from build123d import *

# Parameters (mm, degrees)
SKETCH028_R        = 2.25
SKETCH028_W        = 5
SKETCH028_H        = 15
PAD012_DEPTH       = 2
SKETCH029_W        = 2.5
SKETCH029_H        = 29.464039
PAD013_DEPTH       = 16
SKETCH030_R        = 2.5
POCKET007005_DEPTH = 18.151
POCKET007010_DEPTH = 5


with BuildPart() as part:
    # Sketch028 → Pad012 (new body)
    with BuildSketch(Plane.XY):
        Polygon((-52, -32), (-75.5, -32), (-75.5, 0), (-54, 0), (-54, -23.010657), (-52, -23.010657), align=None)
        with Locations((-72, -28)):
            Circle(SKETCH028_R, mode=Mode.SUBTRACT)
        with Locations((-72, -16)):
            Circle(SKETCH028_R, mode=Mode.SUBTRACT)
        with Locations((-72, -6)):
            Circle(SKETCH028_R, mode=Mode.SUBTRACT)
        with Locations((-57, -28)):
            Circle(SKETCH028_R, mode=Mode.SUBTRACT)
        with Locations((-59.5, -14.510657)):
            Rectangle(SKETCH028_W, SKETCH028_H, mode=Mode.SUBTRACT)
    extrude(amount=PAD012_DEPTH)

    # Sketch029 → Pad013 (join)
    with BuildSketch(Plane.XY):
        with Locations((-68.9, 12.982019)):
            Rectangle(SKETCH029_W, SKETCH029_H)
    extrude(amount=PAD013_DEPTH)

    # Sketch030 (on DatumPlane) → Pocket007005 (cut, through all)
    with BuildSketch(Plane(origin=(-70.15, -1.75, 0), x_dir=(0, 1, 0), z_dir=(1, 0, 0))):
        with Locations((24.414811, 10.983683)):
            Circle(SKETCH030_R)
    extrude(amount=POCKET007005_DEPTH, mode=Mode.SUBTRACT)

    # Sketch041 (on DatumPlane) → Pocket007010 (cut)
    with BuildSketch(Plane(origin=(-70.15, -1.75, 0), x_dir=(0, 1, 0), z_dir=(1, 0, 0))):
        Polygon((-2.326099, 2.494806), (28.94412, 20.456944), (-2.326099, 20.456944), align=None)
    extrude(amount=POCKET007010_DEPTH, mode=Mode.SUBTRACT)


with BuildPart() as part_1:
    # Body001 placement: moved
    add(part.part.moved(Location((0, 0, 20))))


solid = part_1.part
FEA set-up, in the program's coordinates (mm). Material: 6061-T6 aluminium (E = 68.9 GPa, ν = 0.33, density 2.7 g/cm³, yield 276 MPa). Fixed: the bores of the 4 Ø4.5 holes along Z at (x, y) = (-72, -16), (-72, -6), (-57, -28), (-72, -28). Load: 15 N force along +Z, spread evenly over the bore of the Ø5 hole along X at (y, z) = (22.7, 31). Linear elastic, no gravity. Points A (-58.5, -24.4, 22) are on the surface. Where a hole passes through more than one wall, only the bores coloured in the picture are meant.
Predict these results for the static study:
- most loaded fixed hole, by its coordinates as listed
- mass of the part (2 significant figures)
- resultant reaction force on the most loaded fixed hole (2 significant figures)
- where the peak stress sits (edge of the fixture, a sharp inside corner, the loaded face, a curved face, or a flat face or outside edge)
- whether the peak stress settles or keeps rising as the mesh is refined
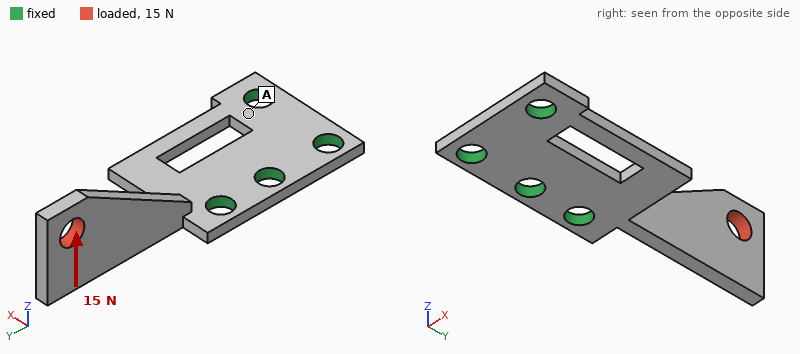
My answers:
(-72, -6)
5.2 g
23 N
a sharp inside corner
keeps rising
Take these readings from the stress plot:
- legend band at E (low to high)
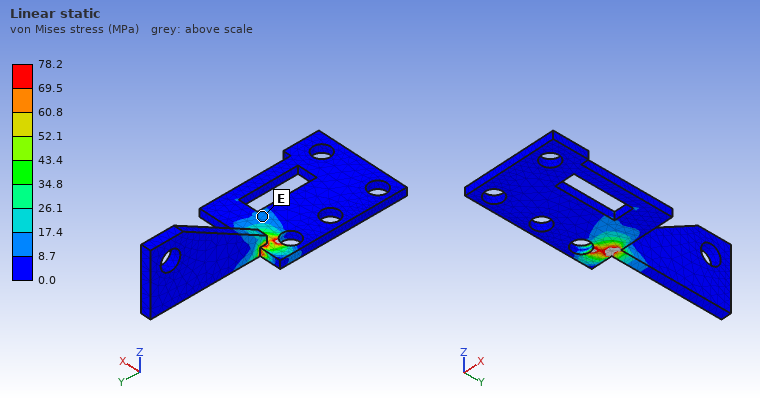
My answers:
8.7 to 17.4 MPa
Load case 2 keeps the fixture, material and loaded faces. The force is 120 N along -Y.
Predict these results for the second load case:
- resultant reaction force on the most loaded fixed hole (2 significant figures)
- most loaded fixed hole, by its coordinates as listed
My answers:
100 N
(-72, -6)
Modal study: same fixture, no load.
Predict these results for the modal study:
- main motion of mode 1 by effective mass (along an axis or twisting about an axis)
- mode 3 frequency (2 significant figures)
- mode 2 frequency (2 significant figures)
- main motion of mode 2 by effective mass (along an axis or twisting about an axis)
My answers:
along Z
5100 Hz
1400 Hz
along X
